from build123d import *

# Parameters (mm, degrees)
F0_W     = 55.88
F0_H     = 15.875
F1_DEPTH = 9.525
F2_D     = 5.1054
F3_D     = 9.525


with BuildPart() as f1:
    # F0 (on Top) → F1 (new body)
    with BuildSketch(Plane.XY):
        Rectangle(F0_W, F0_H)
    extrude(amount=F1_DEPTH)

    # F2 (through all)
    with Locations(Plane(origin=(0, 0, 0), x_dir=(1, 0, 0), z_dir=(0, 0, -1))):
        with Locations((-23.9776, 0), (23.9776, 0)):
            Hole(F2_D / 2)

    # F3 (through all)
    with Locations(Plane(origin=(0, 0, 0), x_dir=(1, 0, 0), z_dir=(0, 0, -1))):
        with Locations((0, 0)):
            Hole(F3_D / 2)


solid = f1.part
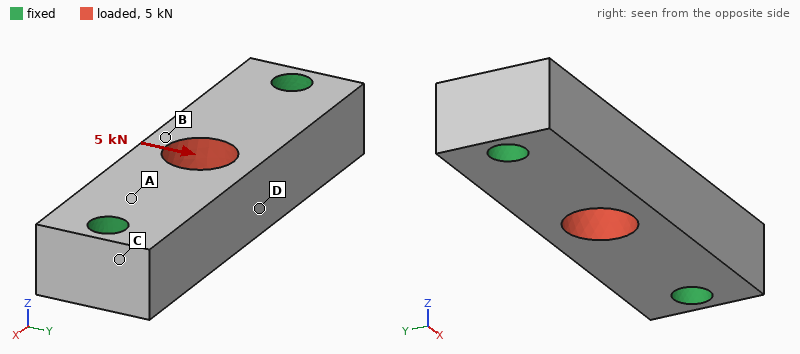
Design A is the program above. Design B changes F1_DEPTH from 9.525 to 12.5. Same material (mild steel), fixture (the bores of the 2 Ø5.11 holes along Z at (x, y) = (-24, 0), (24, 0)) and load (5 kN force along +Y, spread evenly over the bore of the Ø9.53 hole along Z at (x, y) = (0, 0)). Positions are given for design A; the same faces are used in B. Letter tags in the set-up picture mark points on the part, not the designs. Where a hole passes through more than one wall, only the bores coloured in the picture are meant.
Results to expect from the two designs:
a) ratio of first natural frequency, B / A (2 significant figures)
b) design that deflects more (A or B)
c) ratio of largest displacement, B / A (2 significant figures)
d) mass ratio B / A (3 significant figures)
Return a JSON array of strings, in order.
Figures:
["1.2", "A", "0.77", "1.31"]
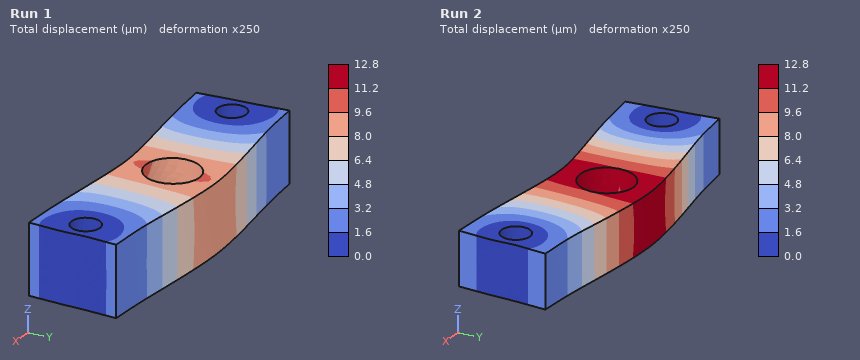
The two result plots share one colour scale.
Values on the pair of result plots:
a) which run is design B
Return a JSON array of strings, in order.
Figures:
["Run 1"]
